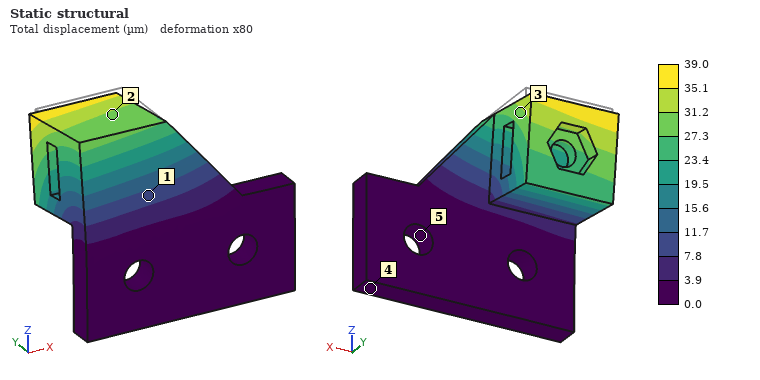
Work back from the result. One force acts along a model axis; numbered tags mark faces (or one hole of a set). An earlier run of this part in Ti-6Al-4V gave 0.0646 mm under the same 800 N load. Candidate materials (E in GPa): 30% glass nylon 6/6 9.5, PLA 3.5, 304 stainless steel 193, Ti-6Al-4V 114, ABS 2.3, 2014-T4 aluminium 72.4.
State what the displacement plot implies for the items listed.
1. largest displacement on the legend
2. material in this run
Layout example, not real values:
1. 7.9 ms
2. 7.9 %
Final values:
1. 39.0 µm
2. 304 stainless steel
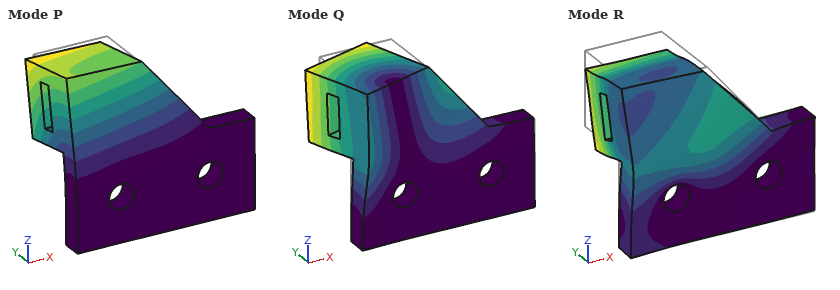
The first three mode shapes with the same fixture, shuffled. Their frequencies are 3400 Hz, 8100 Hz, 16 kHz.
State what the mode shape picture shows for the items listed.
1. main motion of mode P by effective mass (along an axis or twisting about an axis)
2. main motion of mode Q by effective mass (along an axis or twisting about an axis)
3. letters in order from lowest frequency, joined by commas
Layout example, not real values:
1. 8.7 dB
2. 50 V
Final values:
1. along Y
2. along X
3. P, Q, R
